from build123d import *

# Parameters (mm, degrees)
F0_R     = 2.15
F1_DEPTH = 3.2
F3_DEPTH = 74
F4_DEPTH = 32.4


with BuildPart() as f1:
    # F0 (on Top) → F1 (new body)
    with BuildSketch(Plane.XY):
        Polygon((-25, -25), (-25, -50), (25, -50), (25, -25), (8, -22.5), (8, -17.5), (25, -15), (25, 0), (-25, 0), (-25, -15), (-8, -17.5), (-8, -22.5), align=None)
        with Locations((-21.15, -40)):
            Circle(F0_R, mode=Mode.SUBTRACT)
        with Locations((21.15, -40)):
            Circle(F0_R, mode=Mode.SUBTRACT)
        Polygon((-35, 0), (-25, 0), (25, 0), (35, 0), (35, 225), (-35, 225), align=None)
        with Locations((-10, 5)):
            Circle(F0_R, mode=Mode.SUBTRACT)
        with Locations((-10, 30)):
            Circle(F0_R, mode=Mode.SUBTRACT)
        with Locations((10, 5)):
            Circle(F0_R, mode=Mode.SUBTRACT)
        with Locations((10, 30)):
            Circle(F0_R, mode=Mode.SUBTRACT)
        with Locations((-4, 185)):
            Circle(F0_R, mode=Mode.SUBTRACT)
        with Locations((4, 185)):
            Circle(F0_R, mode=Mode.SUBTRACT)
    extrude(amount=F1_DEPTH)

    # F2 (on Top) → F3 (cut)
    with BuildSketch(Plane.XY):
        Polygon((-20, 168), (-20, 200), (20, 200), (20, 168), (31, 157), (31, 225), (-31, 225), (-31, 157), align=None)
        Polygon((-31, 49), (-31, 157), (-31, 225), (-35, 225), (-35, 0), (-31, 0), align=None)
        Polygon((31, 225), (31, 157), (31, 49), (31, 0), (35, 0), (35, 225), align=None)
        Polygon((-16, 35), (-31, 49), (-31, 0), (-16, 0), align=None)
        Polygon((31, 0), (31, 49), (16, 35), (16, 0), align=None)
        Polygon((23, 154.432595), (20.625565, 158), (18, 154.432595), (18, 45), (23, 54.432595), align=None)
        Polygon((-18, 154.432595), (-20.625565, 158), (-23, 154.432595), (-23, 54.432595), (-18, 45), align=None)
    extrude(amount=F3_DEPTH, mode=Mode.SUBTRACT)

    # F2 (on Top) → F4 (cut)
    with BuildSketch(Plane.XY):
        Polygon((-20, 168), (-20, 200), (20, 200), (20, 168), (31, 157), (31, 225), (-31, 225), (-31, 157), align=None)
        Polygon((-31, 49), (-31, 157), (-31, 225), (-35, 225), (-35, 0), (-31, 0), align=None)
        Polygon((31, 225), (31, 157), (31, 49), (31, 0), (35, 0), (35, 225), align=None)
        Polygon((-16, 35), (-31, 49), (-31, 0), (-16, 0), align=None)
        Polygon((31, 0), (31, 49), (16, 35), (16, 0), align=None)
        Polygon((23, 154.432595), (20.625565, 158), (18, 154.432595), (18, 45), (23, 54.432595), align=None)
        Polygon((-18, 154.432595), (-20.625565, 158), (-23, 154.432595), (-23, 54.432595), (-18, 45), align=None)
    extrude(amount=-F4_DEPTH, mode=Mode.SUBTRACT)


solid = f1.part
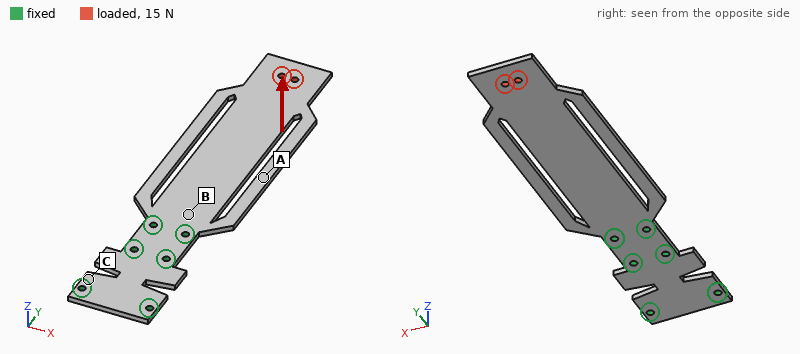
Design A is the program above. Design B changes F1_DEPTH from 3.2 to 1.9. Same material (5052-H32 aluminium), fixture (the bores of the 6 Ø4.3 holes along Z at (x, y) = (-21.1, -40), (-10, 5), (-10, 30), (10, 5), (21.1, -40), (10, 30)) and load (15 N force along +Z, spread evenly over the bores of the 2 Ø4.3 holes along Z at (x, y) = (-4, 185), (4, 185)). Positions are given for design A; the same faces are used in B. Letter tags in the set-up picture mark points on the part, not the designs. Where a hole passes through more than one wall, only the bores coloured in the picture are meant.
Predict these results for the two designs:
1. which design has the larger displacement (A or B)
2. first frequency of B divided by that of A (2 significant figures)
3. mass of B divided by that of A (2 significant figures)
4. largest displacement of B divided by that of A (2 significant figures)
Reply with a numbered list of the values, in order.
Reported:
1. B
2. 0.60
3. 0.59
4. 4.7
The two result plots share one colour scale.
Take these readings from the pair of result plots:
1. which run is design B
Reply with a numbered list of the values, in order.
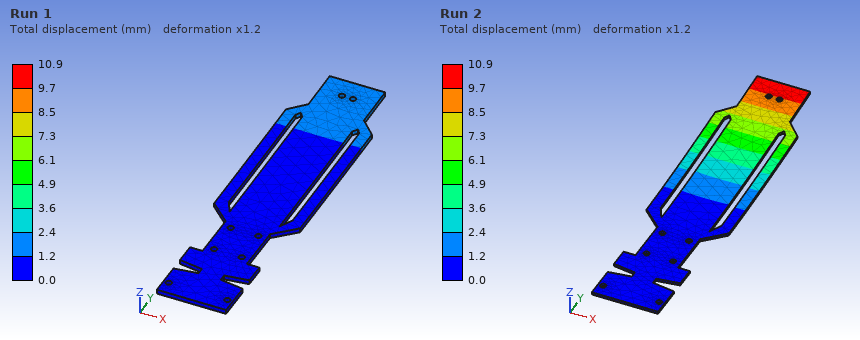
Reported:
1. Run 2
